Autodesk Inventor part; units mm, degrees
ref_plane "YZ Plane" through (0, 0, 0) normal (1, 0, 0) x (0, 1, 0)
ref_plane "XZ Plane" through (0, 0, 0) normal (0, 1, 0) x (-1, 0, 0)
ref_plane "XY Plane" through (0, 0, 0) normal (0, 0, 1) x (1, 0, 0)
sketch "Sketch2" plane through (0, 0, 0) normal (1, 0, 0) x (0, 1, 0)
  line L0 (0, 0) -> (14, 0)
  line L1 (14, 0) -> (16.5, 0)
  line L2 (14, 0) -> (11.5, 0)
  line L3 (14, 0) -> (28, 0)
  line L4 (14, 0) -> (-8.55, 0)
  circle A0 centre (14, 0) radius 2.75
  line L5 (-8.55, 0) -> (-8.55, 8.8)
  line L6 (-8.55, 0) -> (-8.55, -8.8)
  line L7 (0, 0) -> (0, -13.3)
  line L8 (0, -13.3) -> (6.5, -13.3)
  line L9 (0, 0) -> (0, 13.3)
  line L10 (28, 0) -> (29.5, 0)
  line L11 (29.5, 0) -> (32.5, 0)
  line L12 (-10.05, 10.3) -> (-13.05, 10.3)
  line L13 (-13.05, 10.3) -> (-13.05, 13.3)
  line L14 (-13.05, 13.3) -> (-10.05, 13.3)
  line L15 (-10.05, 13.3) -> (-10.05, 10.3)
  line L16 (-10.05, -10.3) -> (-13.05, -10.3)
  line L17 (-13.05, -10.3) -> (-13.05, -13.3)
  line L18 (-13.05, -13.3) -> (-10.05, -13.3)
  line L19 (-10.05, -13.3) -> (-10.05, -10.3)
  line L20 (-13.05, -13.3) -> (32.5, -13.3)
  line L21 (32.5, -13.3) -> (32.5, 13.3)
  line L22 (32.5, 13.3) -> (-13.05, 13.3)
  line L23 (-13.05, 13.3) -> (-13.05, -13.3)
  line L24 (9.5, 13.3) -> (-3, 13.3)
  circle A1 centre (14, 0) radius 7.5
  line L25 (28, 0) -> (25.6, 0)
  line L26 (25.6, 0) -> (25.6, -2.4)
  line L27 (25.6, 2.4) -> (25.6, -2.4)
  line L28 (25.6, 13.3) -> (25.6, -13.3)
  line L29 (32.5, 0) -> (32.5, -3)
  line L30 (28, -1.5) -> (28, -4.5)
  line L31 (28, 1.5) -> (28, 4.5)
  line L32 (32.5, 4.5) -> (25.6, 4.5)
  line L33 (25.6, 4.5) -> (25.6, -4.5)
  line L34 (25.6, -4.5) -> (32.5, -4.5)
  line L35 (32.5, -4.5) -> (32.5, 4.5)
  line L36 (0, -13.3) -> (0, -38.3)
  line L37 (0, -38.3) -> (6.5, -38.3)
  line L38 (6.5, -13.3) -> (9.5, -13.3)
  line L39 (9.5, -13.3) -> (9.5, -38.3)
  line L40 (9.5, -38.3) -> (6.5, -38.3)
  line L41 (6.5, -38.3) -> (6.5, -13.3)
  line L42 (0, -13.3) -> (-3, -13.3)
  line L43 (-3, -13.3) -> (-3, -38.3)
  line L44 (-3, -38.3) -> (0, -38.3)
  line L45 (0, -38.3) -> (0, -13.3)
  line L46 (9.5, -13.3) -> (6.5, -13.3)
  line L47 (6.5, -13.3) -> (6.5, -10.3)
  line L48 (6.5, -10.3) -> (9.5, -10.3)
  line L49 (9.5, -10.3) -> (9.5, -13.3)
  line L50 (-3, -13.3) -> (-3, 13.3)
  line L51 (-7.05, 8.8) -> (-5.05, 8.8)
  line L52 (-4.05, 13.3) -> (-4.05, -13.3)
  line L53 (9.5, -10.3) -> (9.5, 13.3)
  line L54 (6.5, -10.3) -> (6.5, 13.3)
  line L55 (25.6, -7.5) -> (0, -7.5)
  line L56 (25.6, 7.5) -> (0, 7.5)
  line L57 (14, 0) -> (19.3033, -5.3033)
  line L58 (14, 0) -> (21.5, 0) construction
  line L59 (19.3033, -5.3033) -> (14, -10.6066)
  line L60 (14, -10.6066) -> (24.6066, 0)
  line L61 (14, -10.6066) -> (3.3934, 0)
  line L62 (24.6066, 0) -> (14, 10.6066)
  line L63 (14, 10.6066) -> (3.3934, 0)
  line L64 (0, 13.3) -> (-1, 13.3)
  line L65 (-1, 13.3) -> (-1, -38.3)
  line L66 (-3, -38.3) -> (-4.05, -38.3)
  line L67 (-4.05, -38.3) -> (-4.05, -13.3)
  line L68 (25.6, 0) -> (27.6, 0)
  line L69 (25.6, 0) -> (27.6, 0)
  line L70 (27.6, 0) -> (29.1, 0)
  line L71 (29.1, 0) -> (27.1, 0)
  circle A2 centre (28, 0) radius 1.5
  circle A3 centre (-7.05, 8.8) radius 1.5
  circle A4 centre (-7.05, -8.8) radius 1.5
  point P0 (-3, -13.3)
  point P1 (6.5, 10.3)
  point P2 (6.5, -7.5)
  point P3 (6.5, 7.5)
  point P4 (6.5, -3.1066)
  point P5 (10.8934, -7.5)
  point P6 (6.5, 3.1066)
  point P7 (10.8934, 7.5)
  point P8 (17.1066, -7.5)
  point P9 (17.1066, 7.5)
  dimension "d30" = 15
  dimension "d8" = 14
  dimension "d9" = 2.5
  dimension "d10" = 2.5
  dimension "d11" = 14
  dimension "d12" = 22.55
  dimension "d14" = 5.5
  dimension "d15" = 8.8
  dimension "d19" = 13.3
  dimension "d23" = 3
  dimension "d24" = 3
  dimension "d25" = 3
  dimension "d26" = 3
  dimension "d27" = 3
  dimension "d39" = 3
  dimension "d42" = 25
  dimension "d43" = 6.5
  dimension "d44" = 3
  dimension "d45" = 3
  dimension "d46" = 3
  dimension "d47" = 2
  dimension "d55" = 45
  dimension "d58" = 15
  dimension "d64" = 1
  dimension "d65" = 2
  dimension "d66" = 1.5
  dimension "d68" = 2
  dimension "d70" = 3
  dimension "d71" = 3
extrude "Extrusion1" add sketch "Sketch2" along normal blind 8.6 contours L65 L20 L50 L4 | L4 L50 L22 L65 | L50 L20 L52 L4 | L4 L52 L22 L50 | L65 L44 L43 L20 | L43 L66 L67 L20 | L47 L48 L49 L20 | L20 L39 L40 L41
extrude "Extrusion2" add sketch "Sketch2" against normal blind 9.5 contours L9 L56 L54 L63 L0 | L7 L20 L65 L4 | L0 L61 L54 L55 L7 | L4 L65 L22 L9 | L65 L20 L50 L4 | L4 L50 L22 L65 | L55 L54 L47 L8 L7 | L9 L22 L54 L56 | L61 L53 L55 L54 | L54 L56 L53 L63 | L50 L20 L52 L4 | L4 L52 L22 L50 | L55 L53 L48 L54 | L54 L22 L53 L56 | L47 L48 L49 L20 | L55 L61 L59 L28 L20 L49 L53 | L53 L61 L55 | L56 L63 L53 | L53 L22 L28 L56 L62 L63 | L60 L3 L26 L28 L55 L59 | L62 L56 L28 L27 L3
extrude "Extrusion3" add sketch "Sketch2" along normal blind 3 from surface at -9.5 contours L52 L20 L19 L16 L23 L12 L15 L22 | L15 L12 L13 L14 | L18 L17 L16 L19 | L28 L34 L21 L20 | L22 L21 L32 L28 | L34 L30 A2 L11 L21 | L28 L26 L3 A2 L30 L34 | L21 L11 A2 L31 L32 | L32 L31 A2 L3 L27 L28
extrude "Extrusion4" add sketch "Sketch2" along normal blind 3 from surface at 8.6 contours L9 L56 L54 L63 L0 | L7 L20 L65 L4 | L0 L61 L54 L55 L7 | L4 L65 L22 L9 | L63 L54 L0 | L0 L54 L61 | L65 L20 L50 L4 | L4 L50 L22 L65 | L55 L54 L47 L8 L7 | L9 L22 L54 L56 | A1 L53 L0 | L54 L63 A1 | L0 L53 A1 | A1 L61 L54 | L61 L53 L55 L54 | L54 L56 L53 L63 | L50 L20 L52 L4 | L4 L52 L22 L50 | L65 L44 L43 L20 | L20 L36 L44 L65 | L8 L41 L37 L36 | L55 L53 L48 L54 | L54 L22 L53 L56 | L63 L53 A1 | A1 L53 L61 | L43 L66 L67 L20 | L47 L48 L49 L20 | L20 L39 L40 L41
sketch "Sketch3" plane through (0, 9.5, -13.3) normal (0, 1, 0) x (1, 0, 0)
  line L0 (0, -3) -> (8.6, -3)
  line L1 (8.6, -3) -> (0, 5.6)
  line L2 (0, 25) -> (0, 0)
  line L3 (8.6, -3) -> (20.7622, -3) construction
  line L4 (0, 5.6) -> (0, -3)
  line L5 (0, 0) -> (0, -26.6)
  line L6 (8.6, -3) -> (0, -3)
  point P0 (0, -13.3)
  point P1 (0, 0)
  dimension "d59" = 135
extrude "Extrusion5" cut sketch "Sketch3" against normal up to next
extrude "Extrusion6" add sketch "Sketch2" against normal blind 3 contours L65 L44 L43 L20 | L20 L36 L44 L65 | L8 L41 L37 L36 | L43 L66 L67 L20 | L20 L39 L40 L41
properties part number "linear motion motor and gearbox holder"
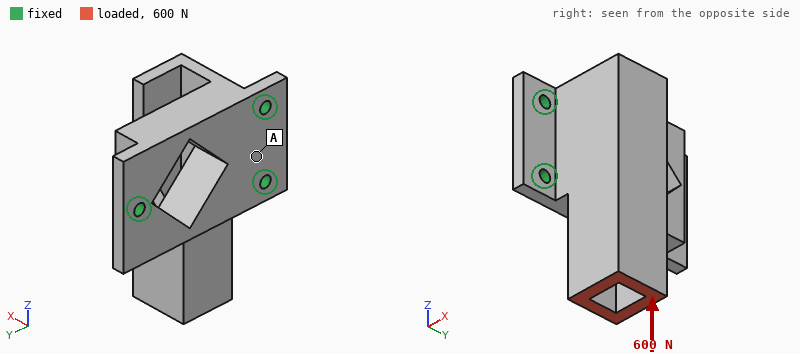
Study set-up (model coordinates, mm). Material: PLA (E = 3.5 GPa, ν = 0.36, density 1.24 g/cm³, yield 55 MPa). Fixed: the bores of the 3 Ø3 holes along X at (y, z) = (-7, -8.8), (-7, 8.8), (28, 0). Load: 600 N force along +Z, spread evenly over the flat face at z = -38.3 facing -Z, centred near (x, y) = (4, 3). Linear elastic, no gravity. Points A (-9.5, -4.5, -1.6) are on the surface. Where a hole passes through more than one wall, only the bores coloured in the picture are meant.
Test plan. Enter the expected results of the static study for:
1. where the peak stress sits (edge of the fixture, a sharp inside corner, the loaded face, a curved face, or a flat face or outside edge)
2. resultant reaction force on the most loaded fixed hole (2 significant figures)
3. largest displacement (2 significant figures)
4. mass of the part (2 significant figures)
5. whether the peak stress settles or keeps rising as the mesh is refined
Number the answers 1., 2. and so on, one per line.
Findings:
1. edge of the fixture
2. 510 N
3. 0.65 mm
4. 14 g
5. keeps rising
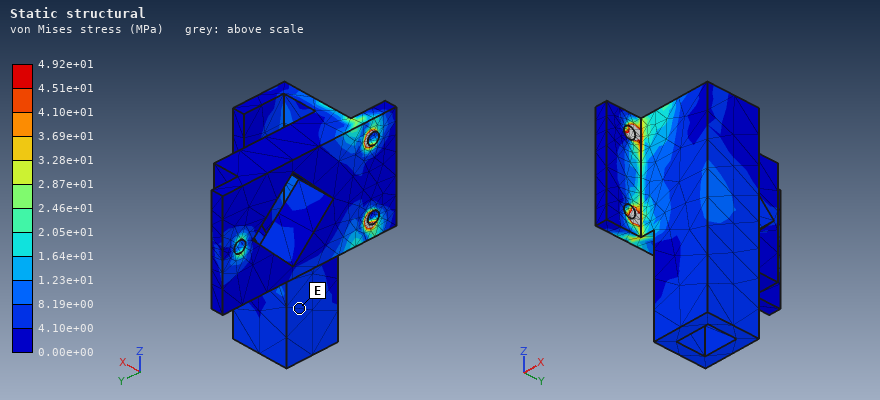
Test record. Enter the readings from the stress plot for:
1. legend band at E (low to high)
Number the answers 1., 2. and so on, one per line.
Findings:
1. 4.10e+00 to 8.19e+00 MPa
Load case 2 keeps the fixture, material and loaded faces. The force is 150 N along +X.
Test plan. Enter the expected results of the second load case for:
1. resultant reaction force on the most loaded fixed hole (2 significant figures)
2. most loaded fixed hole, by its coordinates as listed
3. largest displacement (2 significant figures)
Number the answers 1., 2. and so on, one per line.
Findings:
1. 350 N
2. (-7, -8.8)
3. 0.70 mm
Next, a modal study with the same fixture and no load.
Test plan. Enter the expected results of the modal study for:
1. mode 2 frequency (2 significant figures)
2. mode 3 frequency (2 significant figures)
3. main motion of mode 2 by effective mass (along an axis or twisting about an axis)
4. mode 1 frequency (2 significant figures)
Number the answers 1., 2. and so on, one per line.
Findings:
1. 1700 Hz
2. 2400 Hz
3. along Y
4. 1500 Hz
